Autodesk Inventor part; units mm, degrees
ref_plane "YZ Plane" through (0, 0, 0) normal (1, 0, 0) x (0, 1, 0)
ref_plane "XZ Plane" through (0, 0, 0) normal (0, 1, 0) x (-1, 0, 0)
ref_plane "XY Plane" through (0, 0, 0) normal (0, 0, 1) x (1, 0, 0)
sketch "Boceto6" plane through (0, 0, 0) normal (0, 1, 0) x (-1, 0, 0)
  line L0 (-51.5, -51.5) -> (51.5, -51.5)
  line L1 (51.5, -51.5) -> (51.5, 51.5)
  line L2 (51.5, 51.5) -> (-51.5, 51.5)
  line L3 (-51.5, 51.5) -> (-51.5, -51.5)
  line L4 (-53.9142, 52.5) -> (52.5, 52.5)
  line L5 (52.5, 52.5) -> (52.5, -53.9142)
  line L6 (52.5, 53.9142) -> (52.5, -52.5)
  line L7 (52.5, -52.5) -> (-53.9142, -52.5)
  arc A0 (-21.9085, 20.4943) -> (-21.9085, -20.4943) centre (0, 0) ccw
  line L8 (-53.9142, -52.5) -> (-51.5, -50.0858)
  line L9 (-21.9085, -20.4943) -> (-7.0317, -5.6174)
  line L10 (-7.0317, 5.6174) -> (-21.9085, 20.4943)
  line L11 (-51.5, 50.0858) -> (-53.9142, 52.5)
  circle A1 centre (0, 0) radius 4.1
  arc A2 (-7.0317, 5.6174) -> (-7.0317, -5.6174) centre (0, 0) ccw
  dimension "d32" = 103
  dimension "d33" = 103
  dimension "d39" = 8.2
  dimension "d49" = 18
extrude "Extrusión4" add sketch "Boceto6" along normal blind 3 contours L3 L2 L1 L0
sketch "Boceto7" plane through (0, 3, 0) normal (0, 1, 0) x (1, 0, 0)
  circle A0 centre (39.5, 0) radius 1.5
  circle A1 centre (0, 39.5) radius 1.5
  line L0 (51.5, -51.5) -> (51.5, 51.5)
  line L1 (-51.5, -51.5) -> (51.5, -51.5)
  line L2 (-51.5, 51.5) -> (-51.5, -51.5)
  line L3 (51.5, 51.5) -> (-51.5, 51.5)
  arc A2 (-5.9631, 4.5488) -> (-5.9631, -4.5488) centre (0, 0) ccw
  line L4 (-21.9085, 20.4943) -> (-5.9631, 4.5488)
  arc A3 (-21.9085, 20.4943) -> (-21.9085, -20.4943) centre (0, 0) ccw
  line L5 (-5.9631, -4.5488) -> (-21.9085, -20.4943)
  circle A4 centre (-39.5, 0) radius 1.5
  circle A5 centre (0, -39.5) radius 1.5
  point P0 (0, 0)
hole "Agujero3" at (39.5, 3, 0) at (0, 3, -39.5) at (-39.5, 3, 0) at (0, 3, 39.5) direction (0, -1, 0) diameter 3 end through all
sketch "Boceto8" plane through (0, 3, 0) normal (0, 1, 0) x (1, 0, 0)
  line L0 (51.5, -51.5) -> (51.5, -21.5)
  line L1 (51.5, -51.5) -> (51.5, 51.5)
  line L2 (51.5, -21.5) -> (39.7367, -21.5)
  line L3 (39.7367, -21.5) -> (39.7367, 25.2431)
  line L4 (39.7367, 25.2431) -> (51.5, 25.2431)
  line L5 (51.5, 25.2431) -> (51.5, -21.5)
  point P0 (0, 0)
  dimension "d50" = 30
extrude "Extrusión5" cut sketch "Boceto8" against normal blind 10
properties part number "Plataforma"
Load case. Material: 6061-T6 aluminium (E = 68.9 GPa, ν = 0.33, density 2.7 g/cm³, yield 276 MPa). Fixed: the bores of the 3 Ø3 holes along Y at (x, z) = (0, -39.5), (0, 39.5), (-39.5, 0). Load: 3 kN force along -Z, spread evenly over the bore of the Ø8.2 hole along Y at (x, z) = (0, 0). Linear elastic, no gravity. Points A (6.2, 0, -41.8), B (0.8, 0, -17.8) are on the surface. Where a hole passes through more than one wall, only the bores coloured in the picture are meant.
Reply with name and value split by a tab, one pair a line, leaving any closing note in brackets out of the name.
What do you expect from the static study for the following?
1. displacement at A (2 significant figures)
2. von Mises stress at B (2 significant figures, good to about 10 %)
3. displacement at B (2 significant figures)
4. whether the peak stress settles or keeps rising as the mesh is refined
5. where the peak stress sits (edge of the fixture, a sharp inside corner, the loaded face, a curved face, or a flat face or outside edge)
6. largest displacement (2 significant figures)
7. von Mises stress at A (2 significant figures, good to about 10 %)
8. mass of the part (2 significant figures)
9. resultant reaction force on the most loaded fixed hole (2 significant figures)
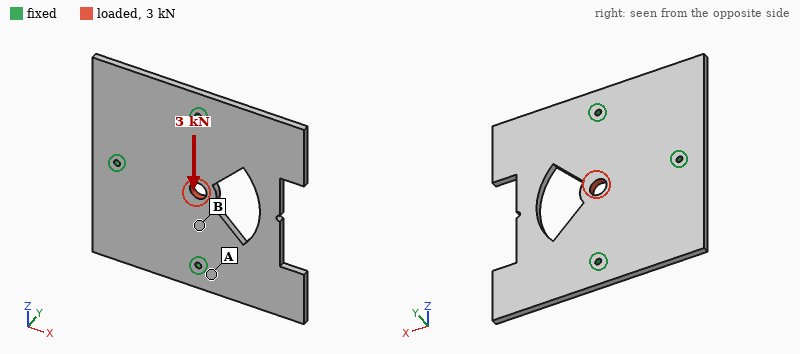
displacement at A	2.9 µm
von Mises stress at B	23 MPa
displacement at B	7.6 µm
whether the peak stress settles or keeps rising as the mesh is refined	keeps rising
where the peak stress sits	edge of the fixture
largest displacement	14 µm
von Mises stress at A	8.6 MPa
mass of the part	76 g
resultant reaction force on the most loaded fixed hole	1.2 kN
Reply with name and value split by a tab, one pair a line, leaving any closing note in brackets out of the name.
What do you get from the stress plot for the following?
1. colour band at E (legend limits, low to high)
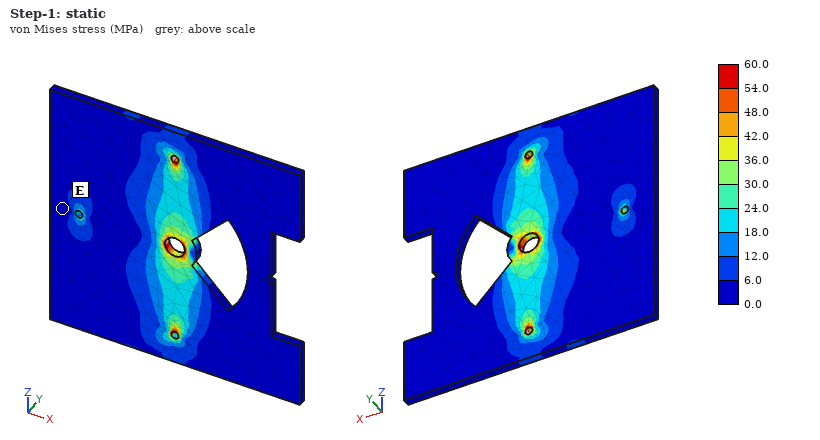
colour band at E	0.0 to 6.0 MPa
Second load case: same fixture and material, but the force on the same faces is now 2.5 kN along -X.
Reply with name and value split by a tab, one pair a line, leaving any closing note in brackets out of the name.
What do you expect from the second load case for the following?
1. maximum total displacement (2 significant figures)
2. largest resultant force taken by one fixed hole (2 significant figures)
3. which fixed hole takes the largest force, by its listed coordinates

maximum total displacement	21 µm
largest resultant force taken by one fixed hole	1.2 kN
which fixed hole takes the largest force, by its listed coordinates	(-39.5, 0)
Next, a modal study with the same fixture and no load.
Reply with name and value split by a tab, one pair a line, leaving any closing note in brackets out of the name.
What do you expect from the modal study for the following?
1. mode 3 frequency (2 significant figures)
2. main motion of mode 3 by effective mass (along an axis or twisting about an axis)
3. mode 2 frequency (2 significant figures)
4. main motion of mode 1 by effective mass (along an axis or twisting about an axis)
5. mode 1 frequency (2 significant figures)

mode 3 frequency	1700 Hz
main motion of mode 3 by effective mass	twisting about X
mode 2 frequency	1200 Hz
main motion of mode 1 by effective mass	along Y
mode 1 frequency	870 Hz
